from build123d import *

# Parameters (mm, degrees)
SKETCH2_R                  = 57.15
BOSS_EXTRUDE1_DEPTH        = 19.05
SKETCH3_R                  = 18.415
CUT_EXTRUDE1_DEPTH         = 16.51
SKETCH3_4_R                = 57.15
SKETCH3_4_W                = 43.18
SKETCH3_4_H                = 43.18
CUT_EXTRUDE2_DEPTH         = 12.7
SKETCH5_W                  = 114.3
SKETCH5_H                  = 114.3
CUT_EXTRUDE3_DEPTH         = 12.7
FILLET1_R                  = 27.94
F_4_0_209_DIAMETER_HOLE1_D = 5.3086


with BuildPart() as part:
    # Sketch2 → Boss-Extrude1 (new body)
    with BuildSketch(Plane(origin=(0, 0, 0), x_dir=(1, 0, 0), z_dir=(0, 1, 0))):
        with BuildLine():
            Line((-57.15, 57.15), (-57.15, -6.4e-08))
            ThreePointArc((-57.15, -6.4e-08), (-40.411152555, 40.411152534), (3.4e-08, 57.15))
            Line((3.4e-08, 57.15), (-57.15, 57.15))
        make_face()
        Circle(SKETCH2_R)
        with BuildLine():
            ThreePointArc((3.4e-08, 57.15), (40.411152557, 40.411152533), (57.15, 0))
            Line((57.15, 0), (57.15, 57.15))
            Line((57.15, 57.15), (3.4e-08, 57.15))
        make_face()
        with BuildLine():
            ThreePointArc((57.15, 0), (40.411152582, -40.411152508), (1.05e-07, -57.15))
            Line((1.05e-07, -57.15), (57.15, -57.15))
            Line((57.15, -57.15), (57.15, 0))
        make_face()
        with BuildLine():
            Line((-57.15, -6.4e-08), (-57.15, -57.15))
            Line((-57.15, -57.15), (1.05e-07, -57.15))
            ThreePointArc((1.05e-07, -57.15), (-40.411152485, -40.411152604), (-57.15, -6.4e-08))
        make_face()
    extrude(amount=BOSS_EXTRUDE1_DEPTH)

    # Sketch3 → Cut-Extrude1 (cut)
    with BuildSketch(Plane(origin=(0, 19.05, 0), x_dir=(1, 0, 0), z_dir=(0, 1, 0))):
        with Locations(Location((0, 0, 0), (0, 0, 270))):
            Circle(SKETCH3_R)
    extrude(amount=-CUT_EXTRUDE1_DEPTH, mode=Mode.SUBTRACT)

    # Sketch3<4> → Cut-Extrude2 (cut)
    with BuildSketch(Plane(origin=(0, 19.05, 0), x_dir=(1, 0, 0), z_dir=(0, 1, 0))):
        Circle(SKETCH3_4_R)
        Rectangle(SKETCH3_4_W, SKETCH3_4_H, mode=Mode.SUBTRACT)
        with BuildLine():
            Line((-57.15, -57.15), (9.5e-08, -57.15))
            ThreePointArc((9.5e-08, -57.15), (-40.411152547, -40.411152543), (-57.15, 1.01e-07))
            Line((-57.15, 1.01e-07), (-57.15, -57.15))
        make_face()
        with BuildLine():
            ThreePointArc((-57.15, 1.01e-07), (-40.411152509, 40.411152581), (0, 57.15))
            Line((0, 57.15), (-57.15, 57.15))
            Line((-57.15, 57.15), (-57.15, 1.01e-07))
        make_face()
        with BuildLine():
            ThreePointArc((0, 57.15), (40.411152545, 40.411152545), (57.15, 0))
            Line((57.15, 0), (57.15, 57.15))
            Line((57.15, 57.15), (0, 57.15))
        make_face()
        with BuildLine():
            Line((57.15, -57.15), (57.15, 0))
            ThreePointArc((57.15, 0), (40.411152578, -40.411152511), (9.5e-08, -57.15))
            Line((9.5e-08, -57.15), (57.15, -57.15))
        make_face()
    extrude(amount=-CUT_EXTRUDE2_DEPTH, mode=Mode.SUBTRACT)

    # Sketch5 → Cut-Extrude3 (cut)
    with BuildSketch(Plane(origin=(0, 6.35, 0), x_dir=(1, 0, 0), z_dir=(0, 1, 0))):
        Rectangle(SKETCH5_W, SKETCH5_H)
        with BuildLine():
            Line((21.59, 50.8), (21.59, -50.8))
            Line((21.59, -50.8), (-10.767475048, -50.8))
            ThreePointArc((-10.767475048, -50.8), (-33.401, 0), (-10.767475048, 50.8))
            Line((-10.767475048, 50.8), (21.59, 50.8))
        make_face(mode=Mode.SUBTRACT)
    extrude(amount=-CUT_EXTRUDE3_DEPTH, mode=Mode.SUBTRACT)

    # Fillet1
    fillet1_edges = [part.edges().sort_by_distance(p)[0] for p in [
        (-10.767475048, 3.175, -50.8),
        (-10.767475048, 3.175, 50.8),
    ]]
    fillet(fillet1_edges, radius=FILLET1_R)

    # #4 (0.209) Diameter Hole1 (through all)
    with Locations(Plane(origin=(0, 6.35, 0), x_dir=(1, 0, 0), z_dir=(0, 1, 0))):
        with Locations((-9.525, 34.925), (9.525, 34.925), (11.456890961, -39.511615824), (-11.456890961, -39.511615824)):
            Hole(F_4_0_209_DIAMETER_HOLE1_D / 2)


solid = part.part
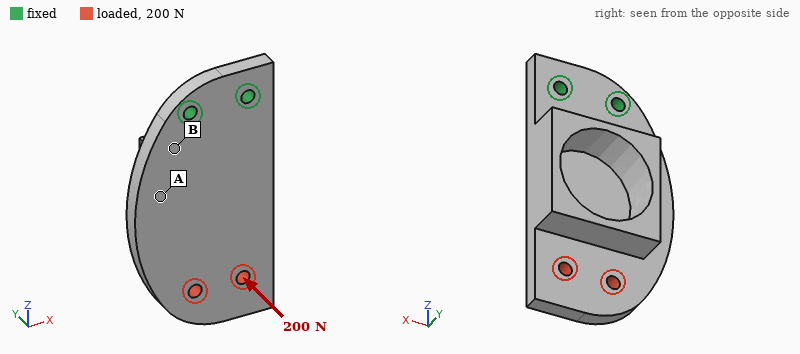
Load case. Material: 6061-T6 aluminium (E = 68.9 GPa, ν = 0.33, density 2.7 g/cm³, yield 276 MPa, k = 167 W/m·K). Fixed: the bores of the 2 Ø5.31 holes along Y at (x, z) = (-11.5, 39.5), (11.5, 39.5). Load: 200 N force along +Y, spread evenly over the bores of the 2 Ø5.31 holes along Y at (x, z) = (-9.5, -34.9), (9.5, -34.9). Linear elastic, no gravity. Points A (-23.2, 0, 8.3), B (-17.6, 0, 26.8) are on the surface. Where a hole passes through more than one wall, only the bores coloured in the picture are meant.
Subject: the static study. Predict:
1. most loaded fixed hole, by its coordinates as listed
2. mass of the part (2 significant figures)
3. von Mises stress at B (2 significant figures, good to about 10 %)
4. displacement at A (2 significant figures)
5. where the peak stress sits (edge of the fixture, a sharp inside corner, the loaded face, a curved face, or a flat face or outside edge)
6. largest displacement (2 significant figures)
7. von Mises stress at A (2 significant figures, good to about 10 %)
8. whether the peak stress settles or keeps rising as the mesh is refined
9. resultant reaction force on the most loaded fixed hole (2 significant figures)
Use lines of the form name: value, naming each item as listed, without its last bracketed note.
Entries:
most loaded fixed hole, by its coordinates as listed: (-11.5, 39.5)
mass of the part: 98 g
von Mises stress at B: 33 MPa
displacement at A: 0.085 mm
where the peak stress sits: edge of the fixture
largest displacement: 0.36 mm
von Mises stress at A: 7.4 MPa
whether the peak stress settles or keeps rising as the mesh is refined: keeps rising
resultant reaction force on the most loaded fixed hole: 110 N
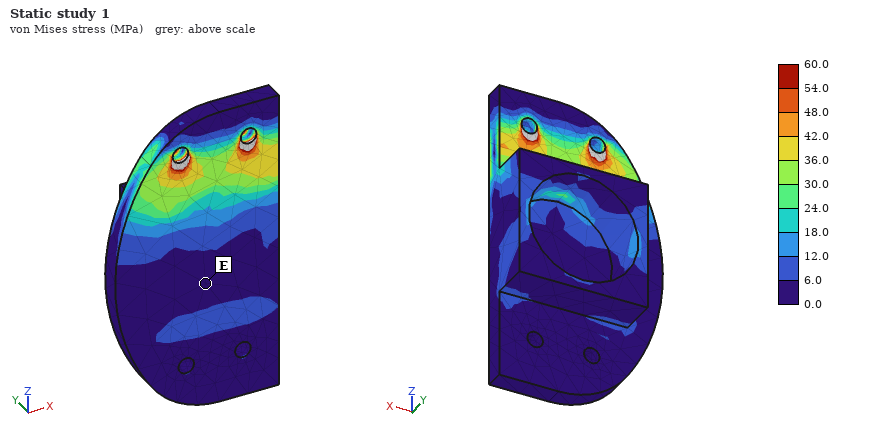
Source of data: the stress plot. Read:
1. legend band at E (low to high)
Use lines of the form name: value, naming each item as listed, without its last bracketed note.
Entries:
legend band at E: 0.0 to 6.0 MPa
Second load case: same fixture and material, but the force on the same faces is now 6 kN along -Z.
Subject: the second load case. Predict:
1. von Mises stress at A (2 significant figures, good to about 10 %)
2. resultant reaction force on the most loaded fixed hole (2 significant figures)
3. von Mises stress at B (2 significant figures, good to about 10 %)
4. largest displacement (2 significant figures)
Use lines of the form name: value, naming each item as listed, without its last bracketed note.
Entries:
von Mises stress at A: 16 MPa
resultant reaction force on the most loaded fixed hole: 3.0 kN
von Mises stress at B: 21 MPa
largest displacement: 45 µm
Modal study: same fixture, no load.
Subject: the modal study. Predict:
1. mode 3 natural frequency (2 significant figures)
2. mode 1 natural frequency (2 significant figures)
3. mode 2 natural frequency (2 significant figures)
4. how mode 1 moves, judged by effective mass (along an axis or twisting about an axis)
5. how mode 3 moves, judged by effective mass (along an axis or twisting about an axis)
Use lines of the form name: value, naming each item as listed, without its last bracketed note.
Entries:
mode 3 natural frequency: 3200 Hz
mode 1 natural frequency: 720 Hz
mode 2 natural frequency: 2400 Hz
how mode 1 moves, judged by effective mass: along Y
how mode 3 moves, judged by effective mass: along X
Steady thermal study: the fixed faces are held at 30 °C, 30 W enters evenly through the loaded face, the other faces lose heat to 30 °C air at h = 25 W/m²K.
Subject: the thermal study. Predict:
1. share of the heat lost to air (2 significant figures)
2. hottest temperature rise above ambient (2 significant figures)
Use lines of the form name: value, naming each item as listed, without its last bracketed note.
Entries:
share of the heat lost to air: 24 %
hottest temperature rise above ambient: 39 K
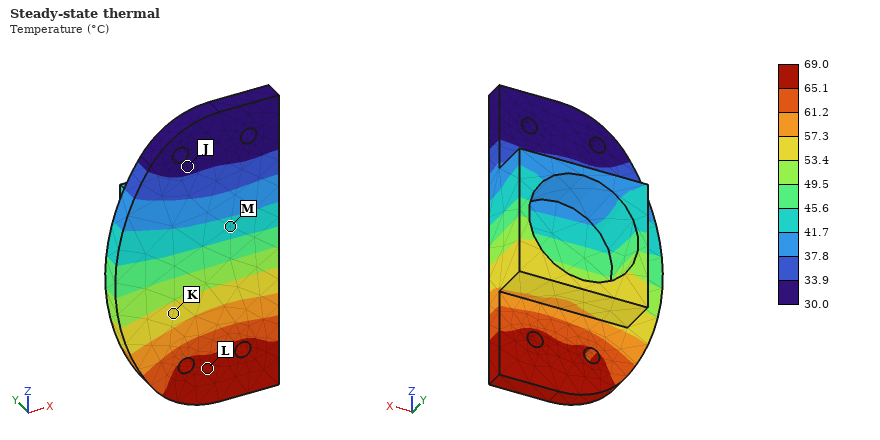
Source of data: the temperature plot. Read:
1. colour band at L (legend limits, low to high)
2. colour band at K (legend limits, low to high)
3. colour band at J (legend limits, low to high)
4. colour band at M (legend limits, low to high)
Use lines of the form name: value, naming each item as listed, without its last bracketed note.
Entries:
colour band at L: 65.1 to 69.0 °C
colour band at K: 53.4 to 57.3 °C
colour band at J: 30.0 to 33.9 °C
colour band at M: 41.7 to 45.6 °C
